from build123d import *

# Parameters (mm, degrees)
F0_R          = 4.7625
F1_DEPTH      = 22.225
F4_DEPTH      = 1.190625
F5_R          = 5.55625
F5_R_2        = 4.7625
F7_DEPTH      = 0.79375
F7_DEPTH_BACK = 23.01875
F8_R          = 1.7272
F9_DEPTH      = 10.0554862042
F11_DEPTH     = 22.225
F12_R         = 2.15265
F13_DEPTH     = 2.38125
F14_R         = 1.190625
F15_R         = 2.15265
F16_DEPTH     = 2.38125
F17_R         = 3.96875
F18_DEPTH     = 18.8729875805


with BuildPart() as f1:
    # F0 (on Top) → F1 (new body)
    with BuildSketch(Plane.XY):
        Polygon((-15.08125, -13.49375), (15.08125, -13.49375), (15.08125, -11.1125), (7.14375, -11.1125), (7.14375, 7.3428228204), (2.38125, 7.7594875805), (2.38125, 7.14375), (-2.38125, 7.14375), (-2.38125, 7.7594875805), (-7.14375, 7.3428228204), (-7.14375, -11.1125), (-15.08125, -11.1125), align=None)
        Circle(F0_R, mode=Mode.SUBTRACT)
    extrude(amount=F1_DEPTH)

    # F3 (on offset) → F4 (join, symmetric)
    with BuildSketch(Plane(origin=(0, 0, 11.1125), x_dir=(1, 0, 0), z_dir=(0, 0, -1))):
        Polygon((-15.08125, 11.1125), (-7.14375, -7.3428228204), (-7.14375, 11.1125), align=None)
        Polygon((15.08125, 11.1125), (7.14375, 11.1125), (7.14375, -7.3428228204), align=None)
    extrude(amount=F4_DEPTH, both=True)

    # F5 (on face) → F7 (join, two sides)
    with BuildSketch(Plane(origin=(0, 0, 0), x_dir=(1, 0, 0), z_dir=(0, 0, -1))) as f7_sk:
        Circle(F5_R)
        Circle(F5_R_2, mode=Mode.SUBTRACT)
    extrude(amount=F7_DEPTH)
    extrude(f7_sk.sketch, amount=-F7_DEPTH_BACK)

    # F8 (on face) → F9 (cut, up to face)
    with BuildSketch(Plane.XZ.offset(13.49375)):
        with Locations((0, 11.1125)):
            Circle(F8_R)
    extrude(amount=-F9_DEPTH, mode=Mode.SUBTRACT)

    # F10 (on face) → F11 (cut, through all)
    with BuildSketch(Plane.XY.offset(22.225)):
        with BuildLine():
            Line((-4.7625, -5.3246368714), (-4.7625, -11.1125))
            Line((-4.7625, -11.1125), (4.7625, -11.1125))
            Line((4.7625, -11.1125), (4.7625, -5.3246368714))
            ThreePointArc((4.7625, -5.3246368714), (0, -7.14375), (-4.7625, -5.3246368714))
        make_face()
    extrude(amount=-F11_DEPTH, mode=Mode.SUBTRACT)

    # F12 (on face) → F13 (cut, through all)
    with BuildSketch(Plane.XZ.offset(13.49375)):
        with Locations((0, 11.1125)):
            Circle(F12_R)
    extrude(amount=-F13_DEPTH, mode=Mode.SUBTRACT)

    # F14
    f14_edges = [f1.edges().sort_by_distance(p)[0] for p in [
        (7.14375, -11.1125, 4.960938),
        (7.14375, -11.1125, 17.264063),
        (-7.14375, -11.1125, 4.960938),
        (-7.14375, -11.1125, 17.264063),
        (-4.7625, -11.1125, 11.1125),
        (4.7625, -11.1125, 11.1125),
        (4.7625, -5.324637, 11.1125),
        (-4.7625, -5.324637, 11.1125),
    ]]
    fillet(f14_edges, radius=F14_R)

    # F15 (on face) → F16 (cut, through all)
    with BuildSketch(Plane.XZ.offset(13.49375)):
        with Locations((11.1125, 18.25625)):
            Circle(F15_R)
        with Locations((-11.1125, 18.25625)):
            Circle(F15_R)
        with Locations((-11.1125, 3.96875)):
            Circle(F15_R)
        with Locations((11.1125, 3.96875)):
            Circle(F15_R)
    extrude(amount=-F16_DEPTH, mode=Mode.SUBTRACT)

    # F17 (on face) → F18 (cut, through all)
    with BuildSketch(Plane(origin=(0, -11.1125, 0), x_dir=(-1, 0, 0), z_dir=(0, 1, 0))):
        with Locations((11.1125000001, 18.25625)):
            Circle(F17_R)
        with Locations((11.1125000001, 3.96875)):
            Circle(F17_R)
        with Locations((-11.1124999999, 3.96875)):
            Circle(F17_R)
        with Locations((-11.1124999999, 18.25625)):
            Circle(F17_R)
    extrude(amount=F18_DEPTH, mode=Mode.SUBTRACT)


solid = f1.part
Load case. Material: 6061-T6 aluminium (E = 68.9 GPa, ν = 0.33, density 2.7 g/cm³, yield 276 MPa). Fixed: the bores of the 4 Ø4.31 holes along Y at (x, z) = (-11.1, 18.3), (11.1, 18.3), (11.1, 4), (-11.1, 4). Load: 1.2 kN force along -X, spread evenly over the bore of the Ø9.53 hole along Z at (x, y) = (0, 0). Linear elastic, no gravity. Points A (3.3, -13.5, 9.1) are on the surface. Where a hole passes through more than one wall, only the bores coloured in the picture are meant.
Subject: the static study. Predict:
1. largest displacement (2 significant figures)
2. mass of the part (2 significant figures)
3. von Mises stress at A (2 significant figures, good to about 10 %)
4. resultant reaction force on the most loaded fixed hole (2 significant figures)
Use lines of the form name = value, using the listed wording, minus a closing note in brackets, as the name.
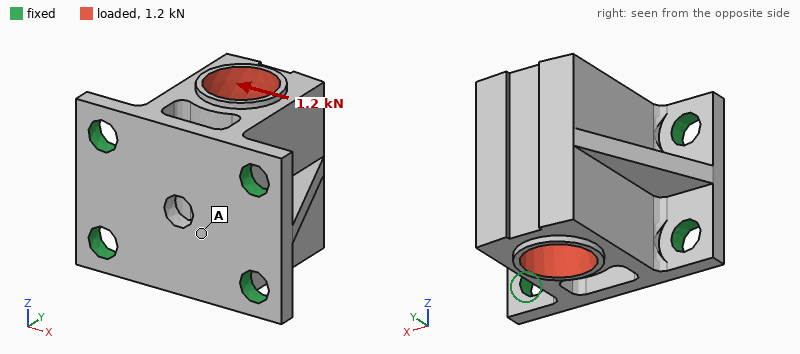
largest displacement = 23 µm
mass of the part = 14 g
von Mises stress at A = 13 MPa
resultant reaction force on the most loaded fixed hole = 470 N
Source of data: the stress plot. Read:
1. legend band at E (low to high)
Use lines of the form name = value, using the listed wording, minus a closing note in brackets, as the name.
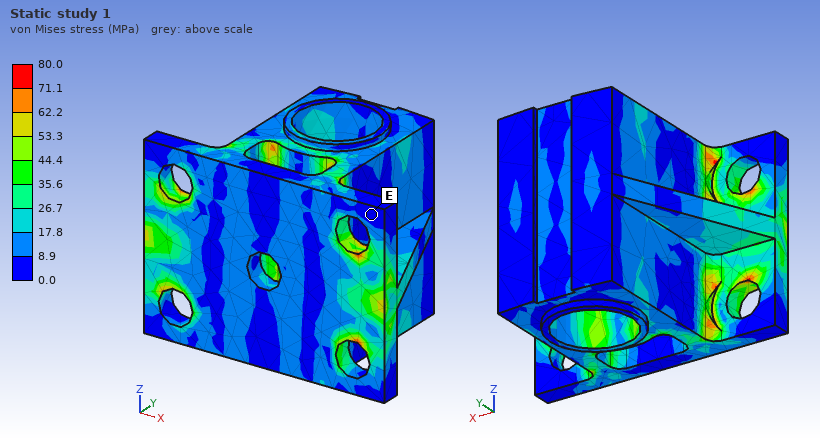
legend band at E = 0.0 to 8.9 MPa
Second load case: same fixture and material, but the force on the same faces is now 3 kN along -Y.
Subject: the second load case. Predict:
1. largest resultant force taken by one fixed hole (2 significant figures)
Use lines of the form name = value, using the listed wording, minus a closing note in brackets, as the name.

largest resultant force taken by one fixed hole = 790 N
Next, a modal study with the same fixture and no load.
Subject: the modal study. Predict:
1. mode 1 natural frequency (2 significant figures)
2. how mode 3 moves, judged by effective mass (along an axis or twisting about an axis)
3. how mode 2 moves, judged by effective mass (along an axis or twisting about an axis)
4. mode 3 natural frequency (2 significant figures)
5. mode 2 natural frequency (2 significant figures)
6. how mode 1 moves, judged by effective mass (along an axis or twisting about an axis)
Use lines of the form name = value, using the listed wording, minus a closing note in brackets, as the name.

mode 1 natural frequency = 12 kHz
how mode 3 moves, judged by effective mass = twisting about Y
how mode 2 moves, judged by effective mass = along X
mode 3 natural frequency = 19 kHz
mode 2 natural frequency = 14 kHz
how mode 1 moves, judged by effective mass = along Z
